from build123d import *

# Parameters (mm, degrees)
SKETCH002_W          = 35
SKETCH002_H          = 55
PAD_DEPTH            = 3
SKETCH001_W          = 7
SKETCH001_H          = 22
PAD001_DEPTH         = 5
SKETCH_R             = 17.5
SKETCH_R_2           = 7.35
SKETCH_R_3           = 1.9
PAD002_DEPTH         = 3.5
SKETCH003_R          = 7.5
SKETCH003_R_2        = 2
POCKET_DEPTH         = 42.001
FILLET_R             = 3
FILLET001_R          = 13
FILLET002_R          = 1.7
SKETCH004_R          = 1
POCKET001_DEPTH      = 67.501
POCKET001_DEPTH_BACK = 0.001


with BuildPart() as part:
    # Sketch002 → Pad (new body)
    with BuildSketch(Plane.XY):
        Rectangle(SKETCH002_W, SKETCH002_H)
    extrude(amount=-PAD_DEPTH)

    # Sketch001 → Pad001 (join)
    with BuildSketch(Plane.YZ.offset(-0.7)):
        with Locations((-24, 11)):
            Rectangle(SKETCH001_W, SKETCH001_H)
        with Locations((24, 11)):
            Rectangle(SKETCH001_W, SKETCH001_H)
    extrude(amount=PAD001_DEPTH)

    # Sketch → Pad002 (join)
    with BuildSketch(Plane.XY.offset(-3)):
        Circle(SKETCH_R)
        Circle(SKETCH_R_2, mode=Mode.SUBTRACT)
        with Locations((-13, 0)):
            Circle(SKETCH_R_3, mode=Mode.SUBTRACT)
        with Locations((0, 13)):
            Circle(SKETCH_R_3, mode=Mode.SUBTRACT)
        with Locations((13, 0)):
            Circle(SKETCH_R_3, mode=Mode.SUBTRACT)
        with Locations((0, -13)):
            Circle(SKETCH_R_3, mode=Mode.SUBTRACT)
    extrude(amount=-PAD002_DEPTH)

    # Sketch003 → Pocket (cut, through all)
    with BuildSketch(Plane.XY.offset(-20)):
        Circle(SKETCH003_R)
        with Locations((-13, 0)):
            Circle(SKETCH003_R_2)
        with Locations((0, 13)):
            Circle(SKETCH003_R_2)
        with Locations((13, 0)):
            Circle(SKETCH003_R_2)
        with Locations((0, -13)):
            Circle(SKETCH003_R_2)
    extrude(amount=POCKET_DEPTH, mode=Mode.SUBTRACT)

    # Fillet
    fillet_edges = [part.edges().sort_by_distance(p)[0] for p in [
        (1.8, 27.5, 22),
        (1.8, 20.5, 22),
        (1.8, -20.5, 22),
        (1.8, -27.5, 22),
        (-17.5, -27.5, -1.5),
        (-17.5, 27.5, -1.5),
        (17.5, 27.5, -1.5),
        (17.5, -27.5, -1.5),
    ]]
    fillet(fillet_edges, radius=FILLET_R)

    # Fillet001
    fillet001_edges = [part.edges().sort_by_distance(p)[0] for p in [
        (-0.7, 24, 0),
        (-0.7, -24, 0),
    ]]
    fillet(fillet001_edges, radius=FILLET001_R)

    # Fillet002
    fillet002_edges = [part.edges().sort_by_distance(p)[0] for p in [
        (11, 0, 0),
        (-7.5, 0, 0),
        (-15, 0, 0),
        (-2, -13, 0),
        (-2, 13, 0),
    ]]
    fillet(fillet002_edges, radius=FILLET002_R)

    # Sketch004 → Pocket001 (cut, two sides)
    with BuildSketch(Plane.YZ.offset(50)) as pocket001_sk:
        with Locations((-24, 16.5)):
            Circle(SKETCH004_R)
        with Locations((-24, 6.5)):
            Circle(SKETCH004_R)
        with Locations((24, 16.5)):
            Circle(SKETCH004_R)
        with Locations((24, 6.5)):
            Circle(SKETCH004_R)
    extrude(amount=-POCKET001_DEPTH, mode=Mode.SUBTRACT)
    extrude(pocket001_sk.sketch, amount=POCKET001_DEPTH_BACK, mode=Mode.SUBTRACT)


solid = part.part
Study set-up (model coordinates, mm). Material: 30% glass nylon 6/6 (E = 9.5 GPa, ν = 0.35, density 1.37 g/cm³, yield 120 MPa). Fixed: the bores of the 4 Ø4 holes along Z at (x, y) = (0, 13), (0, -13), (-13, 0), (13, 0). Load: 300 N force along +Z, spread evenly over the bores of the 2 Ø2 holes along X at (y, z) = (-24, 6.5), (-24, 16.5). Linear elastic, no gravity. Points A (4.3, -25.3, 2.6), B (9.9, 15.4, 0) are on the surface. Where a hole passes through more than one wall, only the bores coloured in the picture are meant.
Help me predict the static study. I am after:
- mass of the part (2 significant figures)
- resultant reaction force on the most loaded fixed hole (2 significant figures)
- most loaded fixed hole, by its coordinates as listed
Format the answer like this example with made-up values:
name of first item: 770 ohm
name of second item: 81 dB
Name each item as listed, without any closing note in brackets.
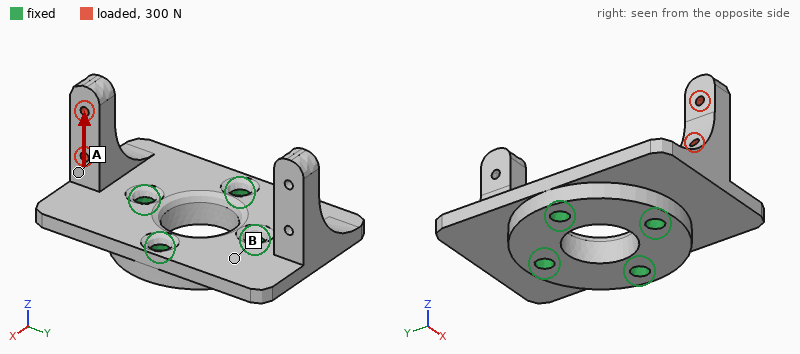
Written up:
mass of the part: 13 g
resultant reaction force on the most loaded fixed hole: 400 N
most loaded fixed hole, by its coordinates as listed: (0, -13)
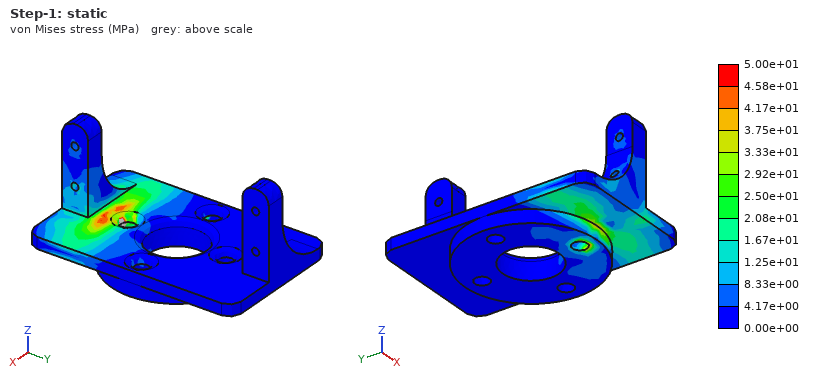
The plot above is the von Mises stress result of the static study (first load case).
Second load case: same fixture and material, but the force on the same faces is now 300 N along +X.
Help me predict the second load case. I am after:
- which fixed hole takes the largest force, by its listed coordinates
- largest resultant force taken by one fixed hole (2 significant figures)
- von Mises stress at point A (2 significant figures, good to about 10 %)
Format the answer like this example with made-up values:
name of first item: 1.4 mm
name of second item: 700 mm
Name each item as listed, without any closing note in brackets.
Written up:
which fixed hole takes the largest force, by its listed coordinates: (0, -13)
largest resultant force taken by one fixed hole: 250 N
von Mises stress at point A: 23 MPa
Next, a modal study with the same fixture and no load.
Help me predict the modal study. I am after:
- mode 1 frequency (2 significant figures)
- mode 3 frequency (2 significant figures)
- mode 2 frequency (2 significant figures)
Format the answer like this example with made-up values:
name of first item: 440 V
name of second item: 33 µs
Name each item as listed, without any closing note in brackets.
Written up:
mode 1 frequency: 2600 Hz
mode 3 frequency: 4000 Hz
mode 2 frequency: 2600 Hz
